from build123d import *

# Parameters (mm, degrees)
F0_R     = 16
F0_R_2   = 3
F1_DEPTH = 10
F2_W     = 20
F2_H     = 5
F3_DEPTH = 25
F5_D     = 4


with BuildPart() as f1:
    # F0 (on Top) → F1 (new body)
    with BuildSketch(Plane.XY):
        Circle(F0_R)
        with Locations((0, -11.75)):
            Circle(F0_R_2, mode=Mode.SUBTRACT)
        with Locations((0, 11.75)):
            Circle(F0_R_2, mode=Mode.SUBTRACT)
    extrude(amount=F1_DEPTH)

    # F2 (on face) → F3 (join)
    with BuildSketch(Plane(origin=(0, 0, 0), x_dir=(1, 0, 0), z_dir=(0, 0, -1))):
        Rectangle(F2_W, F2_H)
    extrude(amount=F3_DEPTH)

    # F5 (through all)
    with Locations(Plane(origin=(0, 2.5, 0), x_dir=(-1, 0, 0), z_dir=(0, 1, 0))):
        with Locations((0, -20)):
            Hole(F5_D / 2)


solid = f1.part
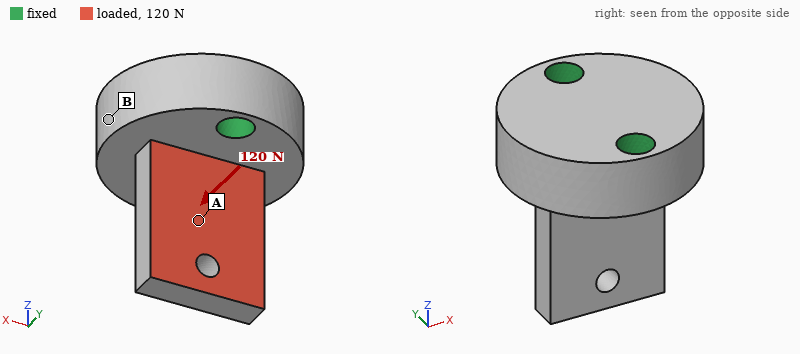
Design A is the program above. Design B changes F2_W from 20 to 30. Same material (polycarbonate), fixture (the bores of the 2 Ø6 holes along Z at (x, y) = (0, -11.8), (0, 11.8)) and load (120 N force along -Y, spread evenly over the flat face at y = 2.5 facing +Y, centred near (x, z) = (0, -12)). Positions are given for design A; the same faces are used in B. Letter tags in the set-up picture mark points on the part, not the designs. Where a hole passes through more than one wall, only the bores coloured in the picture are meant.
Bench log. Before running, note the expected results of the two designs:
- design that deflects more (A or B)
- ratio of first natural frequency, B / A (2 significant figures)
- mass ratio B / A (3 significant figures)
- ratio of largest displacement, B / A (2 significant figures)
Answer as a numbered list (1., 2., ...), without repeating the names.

1. A
2. 0.98
3. 1.13
4. 0.69
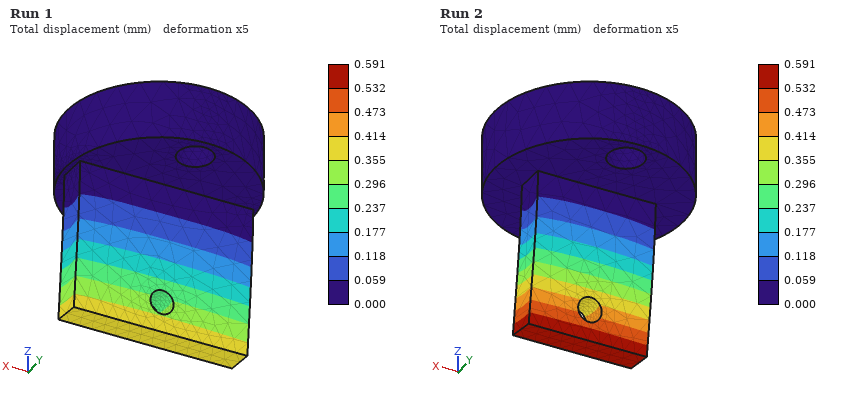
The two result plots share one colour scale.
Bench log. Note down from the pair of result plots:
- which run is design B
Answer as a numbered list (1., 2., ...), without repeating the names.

1. Run 1
